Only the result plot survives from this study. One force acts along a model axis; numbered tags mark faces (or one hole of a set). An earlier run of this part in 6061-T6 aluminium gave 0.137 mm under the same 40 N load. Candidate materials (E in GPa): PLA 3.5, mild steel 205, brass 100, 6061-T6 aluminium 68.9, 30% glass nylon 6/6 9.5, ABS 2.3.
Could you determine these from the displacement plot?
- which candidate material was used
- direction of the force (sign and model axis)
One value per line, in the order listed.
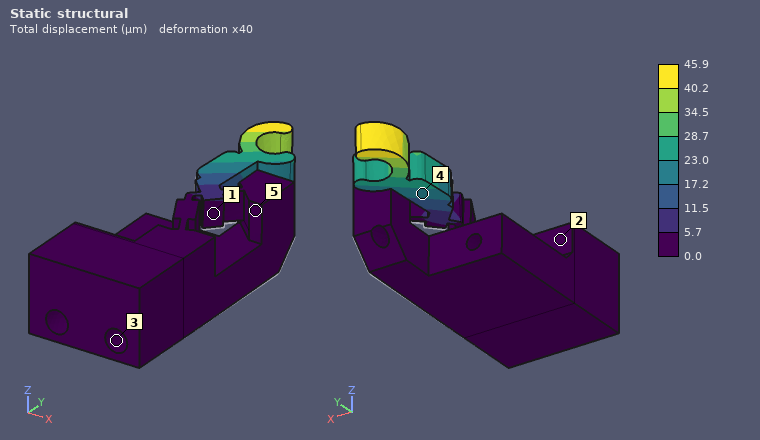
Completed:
mild steel
+Z
